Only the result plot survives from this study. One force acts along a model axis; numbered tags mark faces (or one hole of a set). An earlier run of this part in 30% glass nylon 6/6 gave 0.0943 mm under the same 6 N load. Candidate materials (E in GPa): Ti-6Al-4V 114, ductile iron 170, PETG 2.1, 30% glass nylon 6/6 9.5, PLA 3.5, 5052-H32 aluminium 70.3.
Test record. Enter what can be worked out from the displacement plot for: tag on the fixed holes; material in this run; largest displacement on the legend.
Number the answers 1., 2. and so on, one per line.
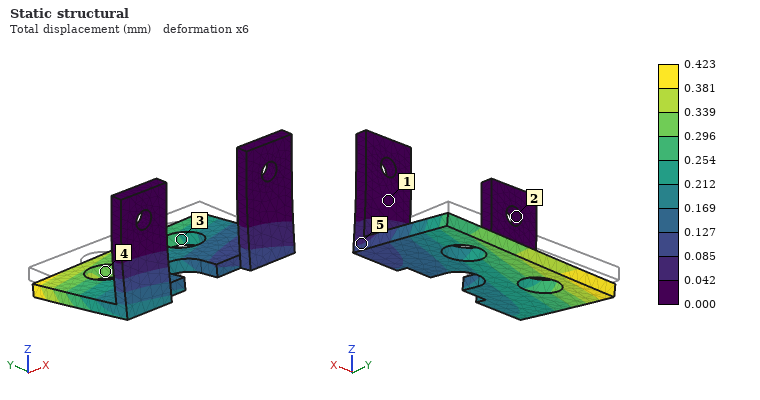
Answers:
1. 2
2. PETG
3. 0.423 mm
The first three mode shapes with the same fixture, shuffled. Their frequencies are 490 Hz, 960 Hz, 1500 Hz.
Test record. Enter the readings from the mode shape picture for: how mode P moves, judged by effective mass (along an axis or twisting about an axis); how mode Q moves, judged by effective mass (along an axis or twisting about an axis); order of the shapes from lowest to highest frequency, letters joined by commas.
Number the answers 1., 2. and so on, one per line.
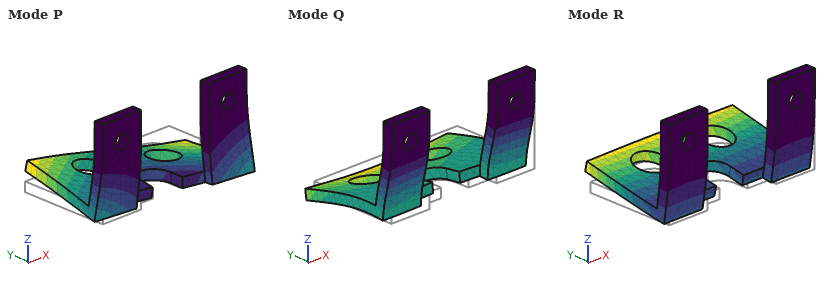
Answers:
1. along X
2. along Y
3. R, P, Q
